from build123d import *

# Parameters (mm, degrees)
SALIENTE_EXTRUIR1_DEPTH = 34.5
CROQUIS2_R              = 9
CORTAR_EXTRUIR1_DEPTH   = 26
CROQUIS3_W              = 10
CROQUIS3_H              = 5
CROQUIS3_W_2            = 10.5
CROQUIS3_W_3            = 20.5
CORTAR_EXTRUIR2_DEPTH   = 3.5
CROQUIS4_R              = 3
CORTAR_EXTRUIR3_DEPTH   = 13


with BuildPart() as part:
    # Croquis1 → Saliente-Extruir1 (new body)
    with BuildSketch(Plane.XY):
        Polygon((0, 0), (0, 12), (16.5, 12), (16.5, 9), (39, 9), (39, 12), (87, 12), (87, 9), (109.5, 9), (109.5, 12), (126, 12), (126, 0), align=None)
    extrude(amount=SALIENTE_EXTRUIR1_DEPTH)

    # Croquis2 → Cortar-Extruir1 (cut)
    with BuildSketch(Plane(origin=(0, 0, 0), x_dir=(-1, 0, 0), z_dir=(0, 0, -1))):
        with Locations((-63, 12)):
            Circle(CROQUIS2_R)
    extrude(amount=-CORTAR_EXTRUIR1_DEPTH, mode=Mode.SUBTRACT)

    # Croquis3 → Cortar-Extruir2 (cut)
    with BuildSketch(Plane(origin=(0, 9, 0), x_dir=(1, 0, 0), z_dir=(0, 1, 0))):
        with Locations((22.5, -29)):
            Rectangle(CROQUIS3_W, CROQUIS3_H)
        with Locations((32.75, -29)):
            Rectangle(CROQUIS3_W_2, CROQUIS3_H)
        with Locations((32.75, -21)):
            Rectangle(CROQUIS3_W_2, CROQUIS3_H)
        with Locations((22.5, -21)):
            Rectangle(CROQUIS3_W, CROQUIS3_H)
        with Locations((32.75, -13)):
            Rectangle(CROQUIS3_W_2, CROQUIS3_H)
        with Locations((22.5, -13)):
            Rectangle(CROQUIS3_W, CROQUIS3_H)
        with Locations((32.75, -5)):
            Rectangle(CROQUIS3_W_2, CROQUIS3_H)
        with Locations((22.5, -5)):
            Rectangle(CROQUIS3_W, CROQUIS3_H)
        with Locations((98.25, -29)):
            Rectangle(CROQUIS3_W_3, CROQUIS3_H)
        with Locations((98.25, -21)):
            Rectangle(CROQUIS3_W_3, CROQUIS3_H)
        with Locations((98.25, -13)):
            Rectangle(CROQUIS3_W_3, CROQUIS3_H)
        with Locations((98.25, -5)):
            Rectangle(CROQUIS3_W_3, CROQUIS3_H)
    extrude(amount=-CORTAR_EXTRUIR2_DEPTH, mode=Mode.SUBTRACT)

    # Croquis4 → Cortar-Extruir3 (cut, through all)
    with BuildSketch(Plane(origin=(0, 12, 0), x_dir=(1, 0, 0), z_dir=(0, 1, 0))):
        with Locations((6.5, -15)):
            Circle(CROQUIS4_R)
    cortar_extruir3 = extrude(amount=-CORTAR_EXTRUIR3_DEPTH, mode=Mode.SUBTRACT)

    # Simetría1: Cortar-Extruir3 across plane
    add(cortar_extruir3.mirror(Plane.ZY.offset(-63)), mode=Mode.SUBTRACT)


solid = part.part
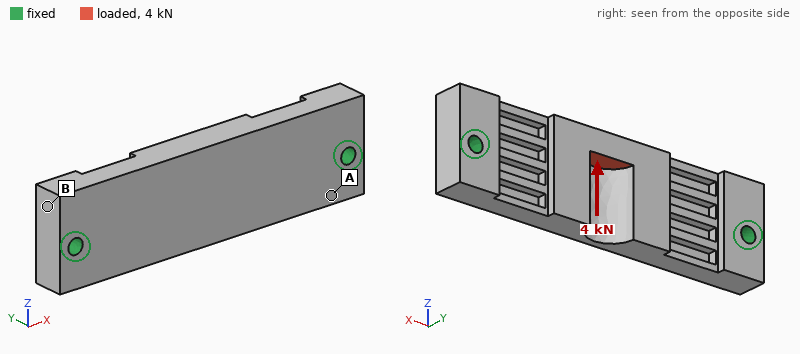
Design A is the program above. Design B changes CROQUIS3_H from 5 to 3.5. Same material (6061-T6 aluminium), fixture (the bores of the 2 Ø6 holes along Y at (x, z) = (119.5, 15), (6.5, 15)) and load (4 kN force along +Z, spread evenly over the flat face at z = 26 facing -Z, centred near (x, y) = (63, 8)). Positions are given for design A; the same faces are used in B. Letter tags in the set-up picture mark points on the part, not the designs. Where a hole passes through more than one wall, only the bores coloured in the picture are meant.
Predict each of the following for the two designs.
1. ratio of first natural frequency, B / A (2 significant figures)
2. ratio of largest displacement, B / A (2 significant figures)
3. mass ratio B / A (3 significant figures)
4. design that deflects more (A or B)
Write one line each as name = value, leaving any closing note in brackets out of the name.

ratio of first natural frequency, B / A = 1.0
ratio of largest displacement, B / A = 0.91
mass ratio B / A = 1.02
design that deflects more = A
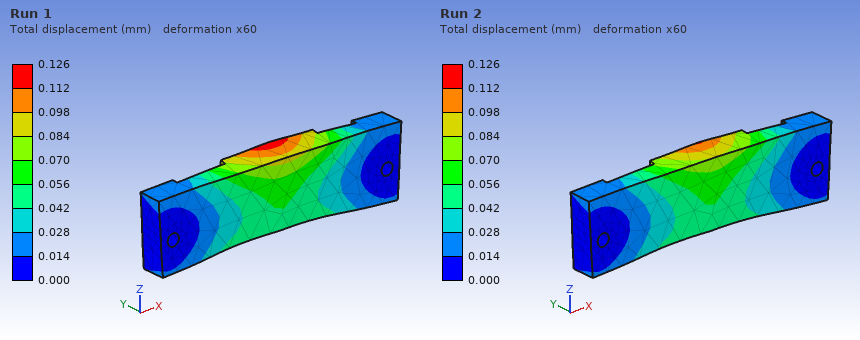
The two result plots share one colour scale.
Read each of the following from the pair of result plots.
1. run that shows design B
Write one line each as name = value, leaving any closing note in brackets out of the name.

run that shows design B = Run 2
